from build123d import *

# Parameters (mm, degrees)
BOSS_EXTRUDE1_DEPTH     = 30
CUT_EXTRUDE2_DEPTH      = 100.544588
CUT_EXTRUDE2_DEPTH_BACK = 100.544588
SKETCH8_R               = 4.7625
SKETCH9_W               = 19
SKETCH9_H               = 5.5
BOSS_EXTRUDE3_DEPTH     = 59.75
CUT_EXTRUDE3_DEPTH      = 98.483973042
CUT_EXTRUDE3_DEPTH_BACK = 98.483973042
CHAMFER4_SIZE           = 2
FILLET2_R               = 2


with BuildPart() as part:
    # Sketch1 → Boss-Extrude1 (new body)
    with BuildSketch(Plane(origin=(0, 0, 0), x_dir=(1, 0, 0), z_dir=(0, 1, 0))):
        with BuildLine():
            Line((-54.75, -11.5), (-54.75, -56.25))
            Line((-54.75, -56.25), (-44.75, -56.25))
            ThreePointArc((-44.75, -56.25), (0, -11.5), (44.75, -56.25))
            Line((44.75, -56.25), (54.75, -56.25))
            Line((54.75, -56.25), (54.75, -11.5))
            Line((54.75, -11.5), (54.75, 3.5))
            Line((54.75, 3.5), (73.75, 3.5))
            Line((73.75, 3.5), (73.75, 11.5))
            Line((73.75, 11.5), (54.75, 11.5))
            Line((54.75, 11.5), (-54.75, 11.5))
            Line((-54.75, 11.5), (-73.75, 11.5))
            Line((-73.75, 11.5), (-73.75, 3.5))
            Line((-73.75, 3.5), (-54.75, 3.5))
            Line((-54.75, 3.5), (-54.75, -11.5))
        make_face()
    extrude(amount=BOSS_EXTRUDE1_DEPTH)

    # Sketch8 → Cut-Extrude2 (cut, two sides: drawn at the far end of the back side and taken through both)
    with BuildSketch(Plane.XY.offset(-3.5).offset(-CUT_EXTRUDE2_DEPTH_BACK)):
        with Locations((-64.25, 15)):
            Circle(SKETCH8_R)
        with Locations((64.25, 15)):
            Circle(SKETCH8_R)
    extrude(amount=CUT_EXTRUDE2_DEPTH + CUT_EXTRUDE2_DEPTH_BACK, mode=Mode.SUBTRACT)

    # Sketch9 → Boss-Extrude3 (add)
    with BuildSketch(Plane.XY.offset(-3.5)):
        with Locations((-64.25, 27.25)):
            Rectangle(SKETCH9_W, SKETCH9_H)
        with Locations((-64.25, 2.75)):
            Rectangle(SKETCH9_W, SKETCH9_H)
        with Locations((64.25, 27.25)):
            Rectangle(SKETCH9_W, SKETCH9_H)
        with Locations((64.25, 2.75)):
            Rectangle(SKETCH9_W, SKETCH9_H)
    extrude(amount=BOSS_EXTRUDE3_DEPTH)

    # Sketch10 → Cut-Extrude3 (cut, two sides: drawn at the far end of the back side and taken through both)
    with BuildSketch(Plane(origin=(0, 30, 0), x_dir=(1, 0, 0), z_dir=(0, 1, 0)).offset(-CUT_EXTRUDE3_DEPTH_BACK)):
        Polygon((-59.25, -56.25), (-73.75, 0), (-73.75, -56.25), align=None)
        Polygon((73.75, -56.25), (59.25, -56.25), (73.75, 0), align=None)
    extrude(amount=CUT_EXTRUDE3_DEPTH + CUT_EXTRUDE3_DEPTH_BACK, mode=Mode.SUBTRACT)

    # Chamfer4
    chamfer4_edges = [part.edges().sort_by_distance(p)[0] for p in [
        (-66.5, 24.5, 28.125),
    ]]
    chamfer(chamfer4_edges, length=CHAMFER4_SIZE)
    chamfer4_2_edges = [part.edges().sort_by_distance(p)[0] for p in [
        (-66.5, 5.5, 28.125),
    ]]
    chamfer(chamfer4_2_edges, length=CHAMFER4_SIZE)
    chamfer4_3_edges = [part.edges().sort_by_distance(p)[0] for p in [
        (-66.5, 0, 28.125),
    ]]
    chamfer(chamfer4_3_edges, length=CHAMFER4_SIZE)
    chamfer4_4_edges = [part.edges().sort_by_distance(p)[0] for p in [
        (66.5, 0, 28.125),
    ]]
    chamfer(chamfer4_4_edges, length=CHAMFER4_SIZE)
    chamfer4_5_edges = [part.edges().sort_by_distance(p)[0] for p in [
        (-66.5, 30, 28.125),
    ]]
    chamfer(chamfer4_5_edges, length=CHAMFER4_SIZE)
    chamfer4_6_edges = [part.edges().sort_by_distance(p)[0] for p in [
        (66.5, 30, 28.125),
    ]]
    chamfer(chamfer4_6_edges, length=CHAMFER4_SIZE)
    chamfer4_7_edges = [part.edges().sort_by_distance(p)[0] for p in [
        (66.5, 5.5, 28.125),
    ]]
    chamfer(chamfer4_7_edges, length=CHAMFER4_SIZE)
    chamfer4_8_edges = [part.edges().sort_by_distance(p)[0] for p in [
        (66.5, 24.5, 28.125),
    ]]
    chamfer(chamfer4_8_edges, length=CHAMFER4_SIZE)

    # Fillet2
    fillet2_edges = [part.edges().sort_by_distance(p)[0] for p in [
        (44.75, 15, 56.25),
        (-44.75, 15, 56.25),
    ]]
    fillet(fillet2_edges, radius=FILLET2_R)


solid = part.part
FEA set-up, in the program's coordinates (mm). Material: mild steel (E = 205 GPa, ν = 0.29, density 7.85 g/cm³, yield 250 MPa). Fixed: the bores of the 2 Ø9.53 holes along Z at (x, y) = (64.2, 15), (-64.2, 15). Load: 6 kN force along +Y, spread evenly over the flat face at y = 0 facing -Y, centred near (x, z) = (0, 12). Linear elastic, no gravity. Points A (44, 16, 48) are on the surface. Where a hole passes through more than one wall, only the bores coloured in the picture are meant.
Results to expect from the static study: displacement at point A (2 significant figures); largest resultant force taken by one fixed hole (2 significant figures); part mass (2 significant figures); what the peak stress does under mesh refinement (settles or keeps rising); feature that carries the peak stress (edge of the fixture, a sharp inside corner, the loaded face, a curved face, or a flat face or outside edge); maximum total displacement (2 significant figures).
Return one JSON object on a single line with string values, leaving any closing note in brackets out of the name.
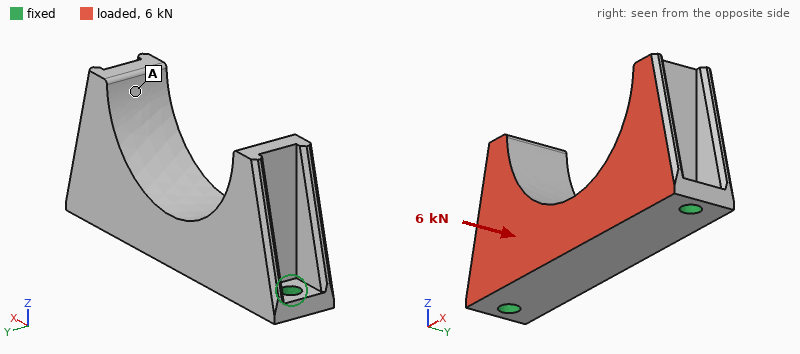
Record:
{"displacement at point A": "42 µm", "largest resultant force taken by one fixed hole": "3.0 kN", "part mass": "1.2 kg", "what the peak stress does under mesh refinement": "keeps rising", "feature that carries the peak stress": "edge of the fixture", "maximum total displacement": "48 µm"}
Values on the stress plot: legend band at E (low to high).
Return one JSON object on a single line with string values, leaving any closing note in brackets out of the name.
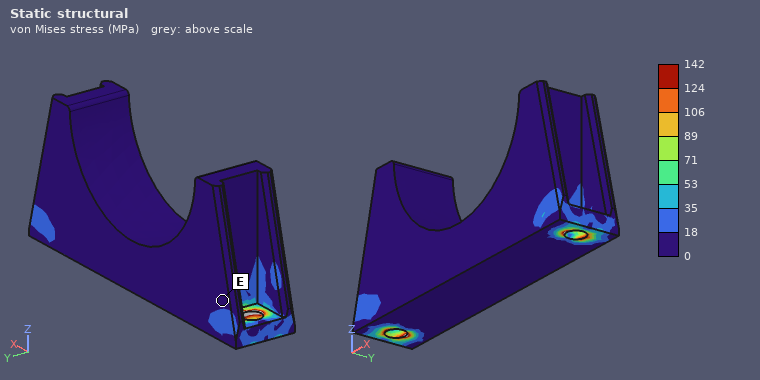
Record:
{"legend band at E": "0 to 18 MPa"}
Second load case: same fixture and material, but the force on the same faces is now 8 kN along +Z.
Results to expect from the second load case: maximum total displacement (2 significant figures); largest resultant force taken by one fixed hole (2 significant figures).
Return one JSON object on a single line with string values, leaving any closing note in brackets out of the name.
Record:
{"maximum total displacement": "47 µm", "largest resultant force taken by one fixed hole": "4.8 kN"}
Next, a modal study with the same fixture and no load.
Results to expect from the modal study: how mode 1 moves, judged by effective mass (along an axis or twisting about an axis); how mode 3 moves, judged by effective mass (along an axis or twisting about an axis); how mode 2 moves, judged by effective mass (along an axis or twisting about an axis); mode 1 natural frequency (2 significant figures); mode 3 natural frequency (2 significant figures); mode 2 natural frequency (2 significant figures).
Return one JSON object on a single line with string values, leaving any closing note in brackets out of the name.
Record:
{"how mode 1 moves, judged by effective mass": "along Y", "how mode 3 moves, judged by effective mass": "twisting about Z", "how mode 2 moves, judged by effective mass": "along Z", "mode 1 natural frequency": "2200 Hz", "mode 3 natural frequency": "3900 Hz", "mode 2 natural frequency": "3700 Hz"}
